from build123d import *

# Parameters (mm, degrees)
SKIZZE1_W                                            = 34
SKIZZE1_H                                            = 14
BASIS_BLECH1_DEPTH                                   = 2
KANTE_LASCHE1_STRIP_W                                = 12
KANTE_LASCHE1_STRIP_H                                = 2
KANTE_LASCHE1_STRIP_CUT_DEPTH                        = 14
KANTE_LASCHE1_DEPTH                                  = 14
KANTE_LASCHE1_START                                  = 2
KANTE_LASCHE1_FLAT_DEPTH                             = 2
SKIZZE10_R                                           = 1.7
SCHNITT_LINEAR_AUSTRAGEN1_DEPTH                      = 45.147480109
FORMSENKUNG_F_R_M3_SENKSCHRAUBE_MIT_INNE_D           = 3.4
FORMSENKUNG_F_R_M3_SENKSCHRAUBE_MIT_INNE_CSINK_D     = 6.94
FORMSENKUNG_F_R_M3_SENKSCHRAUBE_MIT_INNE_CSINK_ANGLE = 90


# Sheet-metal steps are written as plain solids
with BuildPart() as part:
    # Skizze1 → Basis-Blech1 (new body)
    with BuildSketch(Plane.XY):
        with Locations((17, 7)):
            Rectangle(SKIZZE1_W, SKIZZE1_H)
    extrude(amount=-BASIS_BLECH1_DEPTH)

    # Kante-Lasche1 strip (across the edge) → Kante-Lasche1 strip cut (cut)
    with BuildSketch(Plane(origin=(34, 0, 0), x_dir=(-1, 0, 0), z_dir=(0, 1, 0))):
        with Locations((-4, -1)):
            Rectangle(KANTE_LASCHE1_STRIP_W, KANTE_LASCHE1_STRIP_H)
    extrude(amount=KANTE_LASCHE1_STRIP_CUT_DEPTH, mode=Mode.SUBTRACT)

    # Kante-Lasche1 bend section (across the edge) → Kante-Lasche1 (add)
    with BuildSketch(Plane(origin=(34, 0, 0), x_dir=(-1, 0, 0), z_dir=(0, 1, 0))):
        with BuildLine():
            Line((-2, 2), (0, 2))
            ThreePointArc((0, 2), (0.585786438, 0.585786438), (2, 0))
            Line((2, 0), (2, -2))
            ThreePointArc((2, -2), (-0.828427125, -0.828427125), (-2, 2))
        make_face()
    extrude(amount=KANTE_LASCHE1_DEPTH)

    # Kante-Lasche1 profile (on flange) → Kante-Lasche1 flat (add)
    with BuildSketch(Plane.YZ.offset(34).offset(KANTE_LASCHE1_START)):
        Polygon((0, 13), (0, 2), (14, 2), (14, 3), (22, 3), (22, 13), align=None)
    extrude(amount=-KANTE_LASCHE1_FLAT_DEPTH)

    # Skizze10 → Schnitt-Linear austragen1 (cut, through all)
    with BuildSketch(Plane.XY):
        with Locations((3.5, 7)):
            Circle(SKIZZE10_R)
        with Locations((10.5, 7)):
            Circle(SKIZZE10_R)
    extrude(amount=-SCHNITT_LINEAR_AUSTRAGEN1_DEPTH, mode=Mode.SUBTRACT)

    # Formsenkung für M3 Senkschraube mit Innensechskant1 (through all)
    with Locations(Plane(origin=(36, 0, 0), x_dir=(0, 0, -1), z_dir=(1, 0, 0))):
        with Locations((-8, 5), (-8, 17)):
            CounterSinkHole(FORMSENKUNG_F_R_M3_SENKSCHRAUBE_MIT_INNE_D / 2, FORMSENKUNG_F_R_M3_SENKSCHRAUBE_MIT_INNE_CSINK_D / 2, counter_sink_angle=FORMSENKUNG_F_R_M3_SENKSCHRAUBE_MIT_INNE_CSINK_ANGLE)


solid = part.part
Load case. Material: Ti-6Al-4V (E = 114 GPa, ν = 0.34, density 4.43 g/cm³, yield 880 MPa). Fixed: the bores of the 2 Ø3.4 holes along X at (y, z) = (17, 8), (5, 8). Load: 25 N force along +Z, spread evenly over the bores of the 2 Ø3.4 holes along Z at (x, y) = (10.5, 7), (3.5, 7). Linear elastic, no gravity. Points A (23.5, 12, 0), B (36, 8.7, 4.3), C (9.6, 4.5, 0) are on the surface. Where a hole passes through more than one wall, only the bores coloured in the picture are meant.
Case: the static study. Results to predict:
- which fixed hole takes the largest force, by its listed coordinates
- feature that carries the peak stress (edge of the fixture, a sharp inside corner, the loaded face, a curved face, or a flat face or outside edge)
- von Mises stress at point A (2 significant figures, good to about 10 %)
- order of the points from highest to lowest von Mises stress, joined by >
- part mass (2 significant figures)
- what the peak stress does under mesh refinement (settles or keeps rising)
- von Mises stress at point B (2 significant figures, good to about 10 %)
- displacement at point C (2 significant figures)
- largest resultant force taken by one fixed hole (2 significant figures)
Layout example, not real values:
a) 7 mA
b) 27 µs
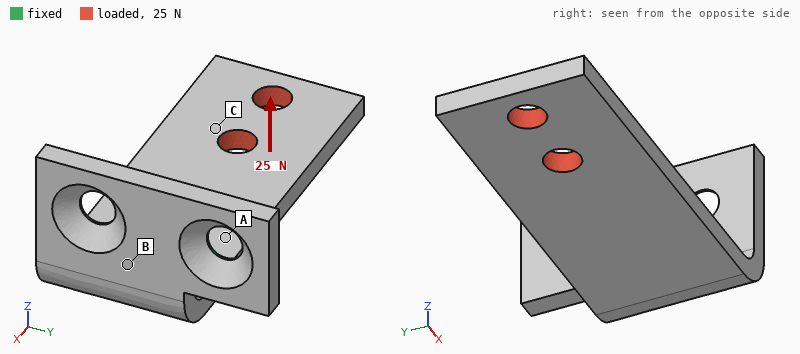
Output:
a) (5, 8)
b) edge of the fixture
c) 44 MPa
d) B > A > C
e) 6.1 g
f) keeps rising
g) 86 MPa
h) 0.34 mm
i) 43 N
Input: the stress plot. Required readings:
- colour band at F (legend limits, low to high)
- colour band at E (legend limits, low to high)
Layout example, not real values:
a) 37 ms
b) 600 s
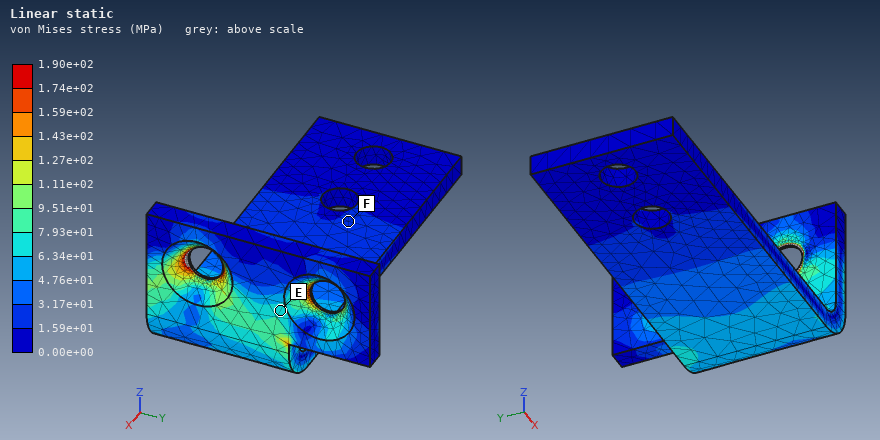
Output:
a) 1.59e+01 to 3.17e+01 MPa
b) 6.34e+01 to 7.93e+01 MPa
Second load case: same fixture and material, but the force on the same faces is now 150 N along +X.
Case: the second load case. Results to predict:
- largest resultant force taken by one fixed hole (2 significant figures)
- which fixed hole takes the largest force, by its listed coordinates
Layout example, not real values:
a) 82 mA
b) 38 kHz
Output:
a) 140 N
b) (5, 8)
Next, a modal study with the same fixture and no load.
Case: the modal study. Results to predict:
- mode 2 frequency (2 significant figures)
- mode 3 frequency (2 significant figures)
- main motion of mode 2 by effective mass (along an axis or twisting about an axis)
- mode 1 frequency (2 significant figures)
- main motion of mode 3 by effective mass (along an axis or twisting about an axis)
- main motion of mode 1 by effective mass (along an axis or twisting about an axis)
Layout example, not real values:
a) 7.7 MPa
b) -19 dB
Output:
a) 1900 Hz
b) 4400 Hz
c) along Y
d) 890 Hz
e) along X
f) along Z
